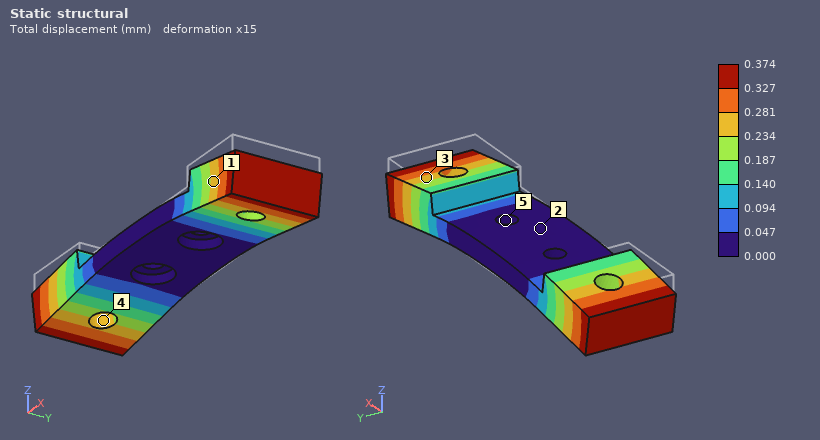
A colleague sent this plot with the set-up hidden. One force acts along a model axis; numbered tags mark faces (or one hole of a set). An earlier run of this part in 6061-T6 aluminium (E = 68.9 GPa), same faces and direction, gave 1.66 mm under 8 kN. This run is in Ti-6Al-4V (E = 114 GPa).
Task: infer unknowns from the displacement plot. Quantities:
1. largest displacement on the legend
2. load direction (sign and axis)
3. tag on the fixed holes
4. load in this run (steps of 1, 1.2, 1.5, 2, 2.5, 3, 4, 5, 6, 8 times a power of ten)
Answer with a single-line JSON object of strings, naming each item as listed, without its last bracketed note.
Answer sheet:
{"largest displacement on the legend": "0.374 mm", "load direction": "-Z", "tag on the fixed holes": "5", "load in this run": "3 kN"}
